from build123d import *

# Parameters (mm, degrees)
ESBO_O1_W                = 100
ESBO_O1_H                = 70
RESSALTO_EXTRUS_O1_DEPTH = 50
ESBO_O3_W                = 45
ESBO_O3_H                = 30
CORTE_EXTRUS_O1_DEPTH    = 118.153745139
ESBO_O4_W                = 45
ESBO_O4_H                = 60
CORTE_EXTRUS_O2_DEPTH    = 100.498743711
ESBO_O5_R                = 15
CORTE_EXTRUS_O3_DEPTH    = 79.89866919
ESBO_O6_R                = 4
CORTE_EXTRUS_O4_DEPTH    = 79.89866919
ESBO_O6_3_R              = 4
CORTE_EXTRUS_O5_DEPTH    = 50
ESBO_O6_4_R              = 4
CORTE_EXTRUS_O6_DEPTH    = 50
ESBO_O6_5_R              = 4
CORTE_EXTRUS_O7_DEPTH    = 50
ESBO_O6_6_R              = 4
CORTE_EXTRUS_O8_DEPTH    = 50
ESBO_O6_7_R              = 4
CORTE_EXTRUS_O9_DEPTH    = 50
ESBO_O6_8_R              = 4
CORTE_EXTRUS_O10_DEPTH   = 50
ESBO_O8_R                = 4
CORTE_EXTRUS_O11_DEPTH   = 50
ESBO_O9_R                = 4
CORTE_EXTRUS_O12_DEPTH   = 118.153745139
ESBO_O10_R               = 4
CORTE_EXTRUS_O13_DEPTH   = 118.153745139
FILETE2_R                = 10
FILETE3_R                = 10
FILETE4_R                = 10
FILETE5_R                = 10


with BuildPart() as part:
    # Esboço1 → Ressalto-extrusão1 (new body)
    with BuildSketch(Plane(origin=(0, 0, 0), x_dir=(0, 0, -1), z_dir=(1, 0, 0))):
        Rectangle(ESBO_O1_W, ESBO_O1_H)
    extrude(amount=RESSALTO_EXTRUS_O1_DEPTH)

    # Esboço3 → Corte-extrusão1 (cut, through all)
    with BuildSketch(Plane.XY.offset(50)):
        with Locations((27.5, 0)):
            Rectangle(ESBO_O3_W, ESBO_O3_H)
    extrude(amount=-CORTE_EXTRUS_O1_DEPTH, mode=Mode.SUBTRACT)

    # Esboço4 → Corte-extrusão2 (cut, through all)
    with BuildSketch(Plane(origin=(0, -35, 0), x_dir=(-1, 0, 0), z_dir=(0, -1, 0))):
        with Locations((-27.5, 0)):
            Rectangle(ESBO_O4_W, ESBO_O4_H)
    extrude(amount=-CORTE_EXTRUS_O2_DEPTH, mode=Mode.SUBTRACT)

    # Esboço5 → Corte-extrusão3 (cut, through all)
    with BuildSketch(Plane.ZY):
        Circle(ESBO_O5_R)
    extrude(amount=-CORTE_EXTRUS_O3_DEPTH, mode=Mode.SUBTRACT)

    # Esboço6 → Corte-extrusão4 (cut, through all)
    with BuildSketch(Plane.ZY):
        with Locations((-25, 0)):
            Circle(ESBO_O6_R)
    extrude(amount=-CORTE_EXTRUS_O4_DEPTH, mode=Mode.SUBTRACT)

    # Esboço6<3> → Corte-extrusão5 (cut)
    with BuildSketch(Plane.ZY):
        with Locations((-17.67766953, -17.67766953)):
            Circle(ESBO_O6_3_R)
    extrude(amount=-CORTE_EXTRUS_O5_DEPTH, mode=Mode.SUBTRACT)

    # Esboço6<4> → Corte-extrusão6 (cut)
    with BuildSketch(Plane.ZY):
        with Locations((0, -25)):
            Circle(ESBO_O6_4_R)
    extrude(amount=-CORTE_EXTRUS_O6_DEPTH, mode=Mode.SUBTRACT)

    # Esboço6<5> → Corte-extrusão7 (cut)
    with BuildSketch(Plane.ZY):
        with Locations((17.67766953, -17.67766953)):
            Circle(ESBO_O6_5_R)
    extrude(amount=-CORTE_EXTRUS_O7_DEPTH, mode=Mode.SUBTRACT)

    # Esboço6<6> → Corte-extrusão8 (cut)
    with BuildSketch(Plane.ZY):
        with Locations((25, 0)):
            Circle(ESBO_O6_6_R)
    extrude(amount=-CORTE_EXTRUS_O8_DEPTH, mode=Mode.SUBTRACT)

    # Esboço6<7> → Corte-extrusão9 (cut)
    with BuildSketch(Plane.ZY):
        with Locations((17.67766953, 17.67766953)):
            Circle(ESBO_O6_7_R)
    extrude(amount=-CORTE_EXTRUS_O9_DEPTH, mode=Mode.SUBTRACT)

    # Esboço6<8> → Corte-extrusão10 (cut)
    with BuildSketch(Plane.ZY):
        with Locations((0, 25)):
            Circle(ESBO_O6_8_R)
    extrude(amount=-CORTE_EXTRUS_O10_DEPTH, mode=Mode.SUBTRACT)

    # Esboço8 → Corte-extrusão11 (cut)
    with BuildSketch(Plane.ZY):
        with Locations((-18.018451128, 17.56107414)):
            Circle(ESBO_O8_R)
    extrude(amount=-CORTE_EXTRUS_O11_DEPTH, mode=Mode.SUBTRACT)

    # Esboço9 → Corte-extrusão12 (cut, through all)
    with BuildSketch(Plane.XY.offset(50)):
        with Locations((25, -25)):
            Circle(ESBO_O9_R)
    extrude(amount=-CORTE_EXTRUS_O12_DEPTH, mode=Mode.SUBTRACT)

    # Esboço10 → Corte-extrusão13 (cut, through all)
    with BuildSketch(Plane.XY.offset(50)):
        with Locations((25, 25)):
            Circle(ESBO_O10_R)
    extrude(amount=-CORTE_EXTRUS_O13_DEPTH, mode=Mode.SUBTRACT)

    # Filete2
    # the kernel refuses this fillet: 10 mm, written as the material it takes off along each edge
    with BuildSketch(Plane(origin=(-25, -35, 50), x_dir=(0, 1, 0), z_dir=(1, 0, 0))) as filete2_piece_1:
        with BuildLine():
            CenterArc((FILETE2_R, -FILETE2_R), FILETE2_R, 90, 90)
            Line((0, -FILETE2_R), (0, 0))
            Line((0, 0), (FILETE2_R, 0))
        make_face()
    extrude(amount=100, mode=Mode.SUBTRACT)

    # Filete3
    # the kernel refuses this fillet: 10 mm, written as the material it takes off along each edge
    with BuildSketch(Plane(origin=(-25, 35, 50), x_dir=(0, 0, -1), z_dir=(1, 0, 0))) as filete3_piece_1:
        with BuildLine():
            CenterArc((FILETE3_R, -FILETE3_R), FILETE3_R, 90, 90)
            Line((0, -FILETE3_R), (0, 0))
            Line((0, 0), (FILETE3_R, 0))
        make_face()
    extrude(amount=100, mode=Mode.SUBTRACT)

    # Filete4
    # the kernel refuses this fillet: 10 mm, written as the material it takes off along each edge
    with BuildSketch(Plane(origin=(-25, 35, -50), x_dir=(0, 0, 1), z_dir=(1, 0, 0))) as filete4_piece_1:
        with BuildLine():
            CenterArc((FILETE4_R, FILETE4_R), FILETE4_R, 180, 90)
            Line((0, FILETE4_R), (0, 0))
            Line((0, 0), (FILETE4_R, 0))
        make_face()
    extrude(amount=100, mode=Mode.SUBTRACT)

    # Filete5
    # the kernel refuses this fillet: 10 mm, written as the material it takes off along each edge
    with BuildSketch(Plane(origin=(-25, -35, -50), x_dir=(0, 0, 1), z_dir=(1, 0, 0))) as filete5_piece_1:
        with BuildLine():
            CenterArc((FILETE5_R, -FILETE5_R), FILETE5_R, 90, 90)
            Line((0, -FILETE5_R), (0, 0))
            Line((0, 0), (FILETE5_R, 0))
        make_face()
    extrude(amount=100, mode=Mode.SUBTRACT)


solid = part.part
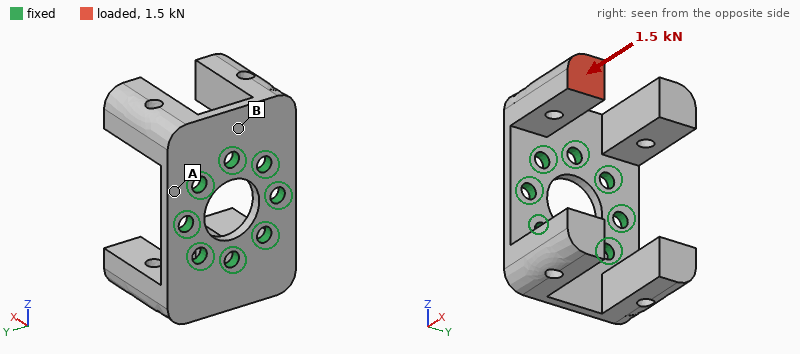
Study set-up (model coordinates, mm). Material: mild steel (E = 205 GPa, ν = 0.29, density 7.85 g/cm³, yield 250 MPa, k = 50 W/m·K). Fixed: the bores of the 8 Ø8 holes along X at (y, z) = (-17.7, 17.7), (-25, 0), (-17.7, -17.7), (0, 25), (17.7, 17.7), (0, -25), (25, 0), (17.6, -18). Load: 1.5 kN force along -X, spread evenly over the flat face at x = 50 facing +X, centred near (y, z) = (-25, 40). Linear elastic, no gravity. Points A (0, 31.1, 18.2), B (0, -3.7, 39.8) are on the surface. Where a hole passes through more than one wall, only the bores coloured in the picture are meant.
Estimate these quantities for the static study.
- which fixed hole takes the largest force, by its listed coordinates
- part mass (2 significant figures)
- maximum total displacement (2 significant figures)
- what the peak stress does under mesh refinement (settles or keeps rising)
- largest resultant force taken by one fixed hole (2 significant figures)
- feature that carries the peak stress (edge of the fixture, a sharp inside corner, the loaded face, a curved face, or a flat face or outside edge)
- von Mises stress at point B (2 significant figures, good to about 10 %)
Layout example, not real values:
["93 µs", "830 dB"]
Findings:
["(-17.7, 17.7)", "730 g", "0.15 mm", "keeps rising", "1.3 kN", "edge of the fixture", "66 MPa"]
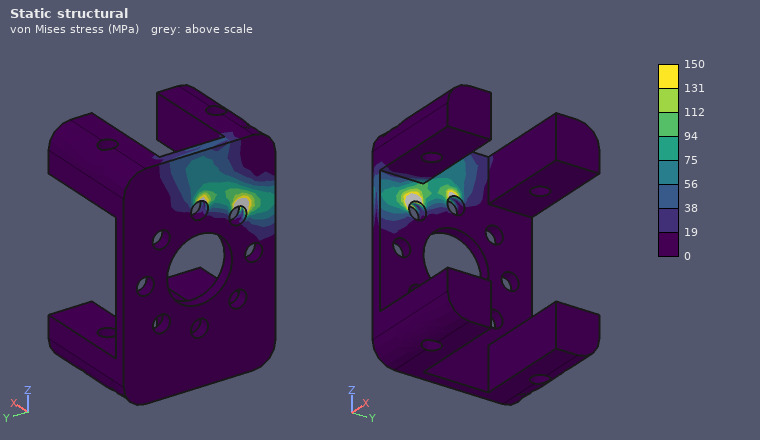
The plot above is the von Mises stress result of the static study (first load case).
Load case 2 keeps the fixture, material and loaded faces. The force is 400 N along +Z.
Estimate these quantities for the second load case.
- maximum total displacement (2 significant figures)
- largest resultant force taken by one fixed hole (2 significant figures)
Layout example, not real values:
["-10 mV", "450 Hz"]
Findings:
["0.13 mm", "500 N"]
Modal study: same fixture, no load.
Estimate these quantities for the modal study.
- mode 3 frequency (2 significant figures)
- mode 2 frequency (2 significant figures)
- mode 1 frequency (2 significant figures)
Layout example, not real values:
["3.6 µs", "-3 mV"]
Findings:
["1200 Hz", "1100 Hz", "1100 Hz"]
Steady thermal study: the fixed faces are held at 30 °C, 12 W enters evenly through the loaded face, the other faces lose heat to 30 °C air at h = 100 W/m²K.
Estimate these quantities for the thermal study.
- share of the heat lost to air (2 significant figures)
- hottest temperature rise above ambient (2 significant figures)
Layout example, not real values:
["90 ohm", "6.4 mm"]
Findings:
["65 %", "30 K"]
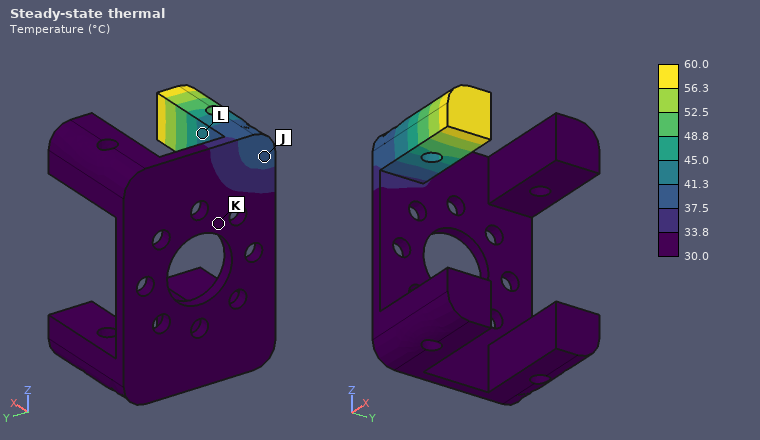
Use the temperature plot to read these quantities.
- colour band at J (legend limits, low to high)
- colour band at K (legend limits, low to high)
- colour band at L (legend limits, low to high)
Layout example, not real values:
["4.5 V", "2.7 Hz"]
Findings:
["37.5 to 41.3 °C", "30.0 to 33.8 °C", "41.3 to 45.0 °C"]
